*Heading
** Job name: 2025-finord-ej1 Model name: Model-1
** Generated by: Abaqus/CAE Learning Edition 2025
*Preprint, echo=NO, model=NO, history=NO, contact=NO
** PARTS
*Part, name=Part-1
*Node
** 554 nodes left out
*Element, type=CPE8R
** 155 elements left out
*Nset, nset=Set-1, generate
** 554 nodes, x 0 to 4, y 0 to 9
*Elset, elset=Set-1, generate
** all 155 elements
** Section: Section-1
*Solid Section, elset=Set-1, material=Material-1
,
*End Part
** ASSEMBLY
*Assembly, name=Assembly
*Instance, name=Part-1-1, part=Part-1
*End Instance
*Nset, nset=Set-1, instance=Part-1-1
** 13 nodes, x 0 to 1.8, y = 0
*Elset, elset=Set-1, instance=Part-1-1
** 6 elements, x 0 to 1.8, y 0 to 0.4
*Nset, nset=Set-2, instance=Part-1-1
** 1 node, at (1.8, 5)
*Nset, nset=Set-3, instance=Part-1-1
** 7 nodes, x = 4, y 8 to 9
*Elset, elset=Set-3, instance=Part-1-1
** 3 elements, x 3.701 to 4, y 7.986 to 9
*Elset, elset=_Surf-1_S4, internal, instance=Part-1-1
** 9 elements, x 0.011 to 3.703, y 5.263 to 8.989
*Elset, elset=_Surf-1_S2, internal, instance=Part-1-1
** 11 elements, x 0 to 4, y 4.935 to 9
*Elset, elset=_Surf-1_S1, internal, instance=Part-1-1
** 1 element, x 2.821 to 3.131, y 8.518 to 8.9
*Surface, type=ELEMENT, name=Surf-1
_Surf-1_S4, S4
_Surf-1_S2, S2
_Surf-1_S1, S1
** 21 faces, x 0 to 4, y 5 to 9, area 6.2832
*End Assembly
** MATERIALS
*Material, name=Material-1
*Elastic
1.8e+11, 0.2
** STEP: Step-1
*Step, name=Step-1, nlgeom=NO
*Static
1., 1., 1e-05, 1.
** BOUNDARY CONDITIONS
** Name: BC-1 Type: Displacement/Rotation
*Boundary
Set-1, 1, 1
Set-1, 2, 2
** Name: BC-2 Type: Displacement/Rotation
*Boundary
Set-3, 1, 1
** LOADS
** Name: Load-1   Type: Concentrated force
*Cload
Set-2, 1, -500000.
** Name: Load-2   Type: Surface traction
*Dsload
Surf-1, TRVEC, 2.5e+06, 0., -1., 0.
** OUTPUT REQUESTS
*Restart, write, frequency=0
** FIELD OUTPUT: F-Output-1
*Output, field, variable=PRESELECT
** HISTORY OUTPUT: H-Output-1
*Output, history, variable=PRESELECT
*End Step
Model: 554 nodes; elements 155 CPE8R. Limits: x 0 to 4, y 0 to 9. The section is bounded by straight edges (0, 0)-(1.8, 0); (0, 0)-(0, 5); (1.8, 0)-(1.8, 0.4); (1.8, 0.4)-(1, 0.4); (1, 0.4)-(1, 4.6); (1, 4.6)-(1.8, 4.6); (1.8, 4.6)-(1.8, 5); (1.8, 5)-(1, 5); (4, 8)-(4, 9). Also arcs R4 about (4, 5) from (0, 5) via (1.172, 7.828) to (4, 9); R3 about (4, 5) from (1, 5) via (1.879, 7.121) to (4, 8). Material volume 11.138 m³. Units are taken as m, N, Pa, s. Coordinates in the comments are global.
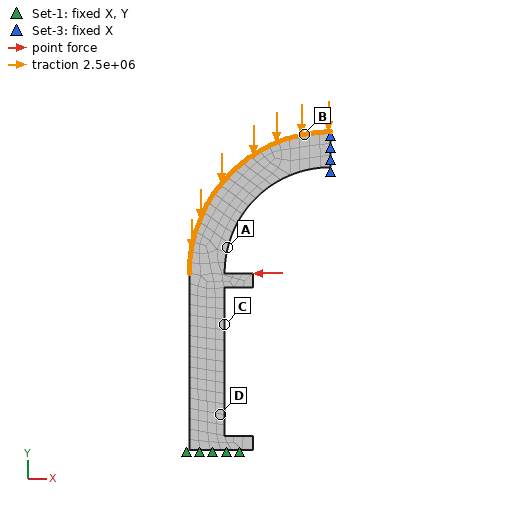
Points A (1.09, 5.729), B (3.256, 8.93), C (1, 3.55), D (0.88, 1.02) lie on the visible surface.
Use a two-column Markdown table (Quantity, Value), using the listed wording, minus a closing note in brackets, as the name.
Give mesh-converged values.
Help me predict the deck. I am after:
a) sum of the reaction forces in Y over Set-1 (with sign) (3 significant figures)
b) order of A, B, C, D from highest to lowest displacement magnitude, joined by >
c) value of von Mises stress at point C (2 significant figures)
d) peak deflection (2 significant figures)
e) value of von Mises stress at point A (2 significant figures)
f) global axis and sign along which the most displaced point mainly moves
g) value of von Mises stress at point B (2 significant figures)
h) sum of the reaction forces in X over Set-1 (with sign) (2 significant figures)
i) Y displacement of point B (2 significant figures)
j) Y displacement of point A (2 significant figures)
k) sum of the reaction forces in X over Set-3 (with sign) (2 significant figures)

| Quantity | Value |
|---|---|
| sum of the reaction forces in Y over Set-1 (with sign) | 1.57e+07 N |
| order of A, B, C, D from highest to lowest displacement magnitude, joined by > | B > A > C > D |
| value of von Mises stress at point C | 2.4e+07 Pa |
| peak deflection | 0.0022 m |
| value of von Mises stress at point A | 4.5e+07 Pa |
| global axis and sign along which the most displaced point mainly moves | -Y |
| value of von Mises stress at point B | 2.7e+07 Pa |
| sum of the reaction forces in X over Set-1 (with sign) | 1.8e+06 N |
| Y displacement of point B | -0.0020 m |
| Y displacement of point A | -6.0e-04 m |
| sum of the reaction forces in X over Set-3 (with sign) | -1.3e+06 N |
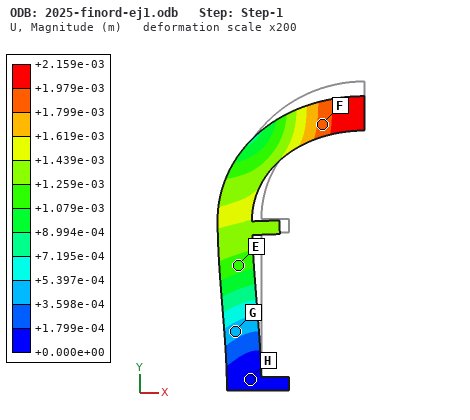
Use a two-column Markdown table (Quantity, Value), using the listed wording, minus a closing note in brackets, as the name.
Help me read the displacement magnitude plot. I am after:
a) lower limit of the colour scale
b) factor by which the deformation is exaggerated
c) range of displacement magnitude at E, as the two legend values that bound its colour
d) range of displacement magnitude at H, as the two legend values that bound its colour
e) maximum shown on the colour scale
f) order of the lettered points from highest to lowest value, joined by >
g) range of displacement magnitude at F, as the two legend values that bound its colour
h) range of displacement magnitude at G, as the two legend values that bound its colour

| Quantity | Value |
|---|---|
| lower limit of the colour scale | +0.000e+00 m |
| factor by which the deformation is exaggerated | 200 |
| range of displacement magnitude at E, as the two legend values that bound its colour | +1.079e-03 to +1.259e-03 m |
| range of displacement magnitude at H, as the two legend values that bound its colour | +0.000e+00 to +1.799e-04 m |
| maximum shown on the colour scale | +2.159e-03 m |
| order of the lettered points from highest to lowest value, joined by > | F > E > G > H |
| range of displacement magnitude at F, as the two legend values that bound its colour | +1.799e-03 to +1.979e-03 m |
| range of displacement magnitude at G, as the two legend values that bound its colour | +3.598e-04 to +5.397e-04 m |
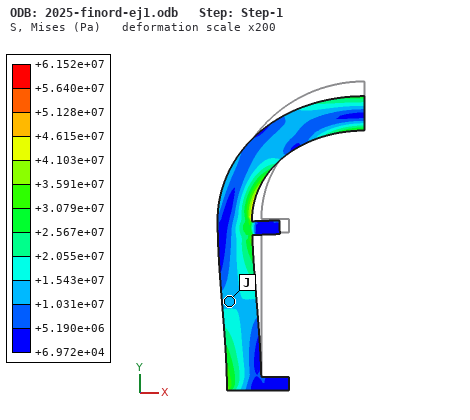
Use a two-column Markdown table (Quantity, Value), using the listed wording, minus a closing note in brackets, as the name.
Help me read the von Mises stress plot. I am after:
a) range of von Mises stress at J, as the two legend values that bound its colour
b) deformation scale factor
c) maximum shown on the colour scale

| Quantity | Value |
|---|---|
| range of von Mises stress at J, as the two legend values that bound its colour | +1.031e+07 to +1.543e+07 Pa |
| deformation scale factor | 200 |
| maximum shown on the colour scale | +6.152e+07 Pa |
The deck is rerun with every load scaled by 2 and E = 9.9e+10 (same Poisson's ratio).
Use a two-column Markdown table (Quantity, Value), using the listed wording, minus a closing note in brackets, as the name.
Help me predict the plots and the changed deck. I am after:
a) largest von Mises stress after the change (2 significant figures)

| Quantity | Value |
|---|---|
| largest von Mises stress after the change | 1.2e+08 Pa |
